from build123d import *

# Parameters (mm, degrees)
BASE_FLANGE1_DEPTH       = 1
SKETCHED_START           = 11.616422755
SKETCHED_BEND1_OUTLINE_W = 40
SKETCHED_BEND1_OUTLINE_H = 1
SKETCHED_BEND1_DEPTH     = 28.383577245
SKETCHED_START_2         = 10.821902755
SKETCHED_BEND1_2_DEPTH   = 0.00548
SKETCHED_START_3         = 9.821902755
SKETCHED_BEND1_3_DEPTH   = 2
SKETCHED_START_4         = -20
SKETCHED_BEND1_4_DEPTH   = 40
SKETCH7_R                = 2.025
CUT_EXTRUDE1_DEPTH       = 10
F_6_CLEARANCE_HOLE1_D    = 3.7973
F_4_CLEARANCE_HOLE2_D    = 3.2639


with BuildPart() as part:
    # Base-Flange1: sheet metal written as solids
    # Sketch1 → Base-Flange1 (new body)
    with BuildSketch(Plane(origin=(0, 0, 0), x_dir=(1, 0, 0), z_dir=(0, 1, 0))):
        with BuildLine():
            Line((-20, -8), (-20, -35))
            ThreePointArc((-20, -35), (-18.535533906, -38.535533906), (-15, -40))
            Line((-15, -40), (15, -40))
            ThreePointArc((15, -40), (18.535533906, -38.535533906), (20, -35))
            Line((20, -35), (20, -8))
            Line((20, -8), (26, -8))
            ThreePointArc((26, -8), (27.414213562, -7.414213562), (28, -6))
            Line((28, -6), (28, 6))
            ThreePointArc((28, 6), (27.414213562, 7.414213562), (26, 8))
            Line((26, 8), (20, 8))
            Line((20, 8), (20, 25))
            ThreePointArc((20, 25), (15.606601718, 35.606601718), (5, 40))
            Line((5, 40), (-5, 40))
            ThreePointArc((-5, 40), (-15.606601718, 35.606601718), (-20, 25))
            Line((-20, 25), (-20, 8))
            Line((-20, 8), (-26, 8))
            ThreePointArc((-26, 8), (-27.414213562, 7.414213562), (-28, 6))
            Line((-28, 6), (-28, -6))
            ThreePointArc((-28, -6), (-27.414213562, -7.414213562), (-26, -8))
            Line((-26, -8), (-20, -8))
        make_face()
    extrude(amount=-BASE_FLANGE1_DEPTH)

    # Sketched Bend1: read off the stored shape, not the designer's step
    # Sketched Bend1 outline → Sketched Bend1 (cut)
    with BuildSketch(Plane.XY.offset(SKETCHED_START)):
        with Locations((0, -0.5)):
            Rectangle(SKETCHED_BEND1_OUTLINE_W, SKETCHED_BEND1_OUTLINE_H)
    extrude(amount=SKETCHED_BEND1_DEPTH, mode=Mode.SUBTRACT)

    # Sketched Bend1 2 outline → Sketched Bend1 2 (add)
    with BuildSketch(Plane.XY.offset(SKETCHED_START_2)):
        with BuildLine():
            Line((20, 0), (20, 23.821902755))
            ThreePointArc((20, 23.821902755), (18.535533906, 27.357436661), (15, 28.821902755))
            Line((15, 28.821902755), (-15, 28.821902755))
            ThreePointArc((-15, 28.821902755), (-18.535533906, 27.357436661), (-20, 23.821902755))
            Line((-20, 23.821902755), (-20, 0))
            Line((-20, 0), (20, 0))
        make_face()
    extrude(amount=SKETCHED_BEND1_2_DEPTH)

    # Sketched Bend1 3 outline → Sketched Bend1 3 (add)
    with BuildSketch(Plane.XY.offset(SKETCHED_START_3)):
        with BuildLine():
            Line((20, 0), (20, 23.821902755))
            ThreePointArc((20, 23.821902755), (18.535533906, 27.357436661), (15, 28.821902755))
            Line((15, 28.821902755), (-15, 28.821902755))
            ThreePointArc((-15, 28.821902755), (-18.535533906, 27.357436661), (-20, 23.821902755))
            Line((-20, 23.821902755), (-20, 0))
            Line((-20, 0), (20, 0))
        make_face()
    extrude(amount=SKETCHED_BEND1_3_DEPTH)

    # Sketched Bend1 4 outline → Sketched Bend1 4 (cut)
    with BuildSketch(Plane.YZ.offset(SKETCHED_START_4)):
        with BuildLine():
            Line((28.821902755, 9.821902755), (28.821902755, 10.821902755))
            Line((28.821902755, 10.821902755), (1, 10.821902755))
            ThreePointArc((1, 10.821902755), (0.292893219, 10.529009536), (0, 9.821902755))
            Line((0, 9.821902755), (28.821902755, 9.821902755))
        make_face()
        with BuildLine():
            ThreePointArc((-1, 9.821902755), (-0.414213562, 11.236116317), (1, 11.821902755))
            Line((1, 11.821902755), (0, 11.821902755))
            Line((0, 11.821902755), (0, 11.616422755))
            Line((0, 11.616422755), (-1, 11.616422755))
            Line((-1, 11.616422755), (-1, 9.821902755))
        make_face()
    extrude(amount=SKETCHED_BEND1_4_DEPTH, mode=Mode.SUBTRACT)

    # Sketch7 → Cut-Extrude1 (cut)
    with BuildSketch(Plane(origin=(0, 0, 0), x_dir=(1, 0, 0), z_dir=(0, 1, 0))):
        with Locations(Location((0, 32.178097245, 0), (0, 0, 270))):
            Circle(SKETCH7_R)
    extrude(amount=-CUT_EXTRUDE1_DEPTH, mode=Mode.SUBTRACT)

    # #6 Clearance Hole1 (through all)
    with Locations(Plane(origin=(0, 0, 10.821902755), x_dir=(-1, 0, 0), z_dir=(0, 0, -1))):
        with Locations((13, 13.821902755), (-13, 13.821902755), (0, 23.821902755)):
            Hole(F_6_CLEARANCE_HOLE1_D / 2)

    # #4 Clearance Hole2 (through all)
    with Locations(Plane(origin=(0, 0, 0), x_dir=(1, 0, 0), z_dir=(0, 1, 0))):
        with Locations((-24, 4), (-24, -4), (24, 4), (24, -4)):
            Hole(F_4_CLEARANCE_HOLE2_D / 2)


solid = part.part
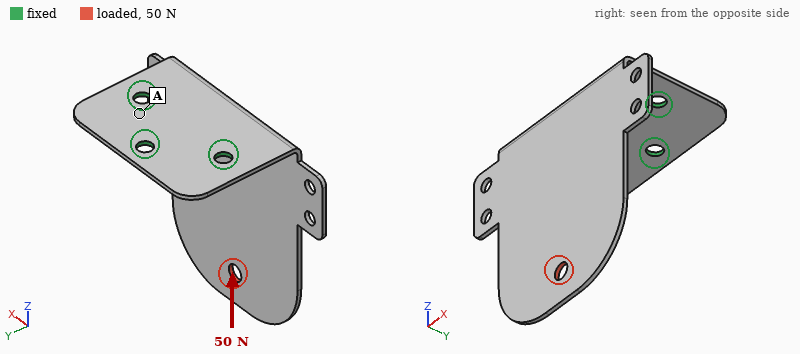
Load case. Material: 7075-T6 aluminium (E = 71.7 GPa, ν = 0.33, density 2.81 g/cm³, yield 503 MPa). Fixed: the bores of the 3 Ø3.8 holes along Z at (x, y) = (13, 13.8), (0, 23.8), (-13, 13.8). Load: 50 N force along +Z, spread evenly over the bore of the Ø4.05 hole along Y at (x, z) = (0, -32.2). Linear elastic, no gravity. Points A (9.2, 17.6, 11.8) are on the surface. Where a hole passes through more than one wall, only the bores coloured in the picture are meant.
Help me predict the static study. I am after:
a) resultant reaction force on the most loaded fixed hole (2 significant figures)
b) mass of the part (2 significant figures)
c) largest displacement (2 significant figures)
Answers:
30 N
9.2 g
0.97 mm
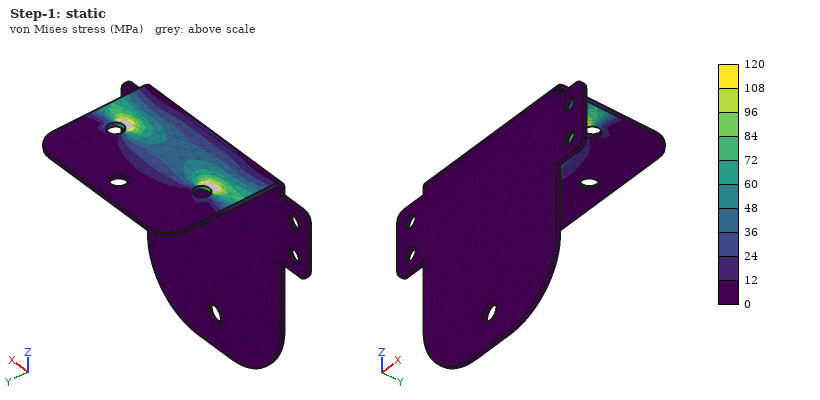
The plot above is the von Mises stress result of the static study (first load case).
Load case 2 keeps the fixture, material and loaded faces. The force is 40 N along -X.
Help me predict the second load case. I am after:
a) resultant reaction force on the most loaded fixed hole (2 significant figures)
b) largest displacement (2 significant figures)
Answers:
68 N
0.88 mm
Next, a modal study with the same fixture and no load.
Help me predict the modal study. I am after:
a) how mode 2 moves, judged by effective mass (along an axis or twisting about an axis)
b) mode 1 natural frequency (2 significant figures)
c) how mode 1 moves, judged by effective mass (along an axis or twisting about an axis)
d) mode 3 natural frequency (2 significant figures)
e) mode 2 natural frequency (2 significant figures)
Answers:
along X
250 Hz
along Y
1100 Hz
650 Hz
